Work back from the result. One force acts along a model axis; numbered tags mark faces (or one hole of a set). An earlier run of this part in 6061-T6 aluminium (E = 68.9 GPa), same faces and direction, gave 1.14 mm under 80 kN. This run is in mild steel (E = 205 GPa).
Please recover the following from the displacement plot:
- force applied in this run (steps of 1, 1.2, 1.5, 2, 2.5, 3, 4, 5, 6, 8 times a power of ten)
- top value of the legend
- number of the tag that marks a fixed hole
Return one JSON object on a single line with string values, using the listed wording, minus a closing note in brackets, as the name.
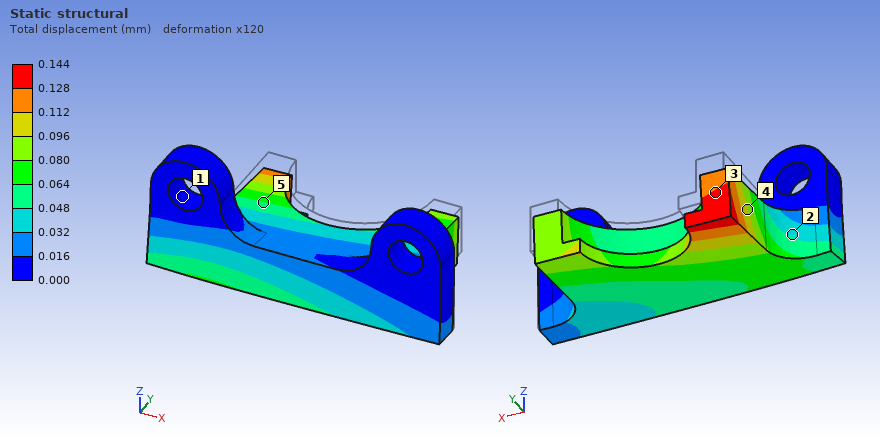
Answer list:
{"force applied in this run": "30 kN", "top value of the legend": "0.144 mm", "number of the tag that marks a fixed hole": "1"}
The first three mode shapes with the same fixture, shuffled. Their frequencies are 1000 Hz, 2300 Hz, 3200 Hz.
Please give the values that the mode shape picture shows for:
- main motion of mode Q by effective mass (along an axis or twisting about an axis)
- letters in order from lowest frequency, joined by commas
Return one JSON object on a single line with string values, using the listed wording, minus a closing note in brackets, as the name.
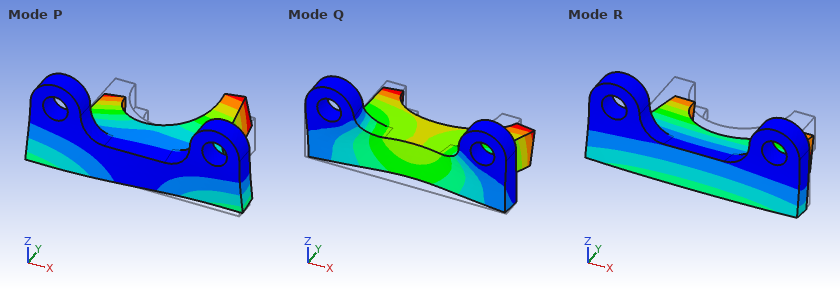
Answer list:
{"main motion of mode Q by effective mass": "along Y", "letters in order from lowest frequency, joined by commas": "R, P, Q"}
